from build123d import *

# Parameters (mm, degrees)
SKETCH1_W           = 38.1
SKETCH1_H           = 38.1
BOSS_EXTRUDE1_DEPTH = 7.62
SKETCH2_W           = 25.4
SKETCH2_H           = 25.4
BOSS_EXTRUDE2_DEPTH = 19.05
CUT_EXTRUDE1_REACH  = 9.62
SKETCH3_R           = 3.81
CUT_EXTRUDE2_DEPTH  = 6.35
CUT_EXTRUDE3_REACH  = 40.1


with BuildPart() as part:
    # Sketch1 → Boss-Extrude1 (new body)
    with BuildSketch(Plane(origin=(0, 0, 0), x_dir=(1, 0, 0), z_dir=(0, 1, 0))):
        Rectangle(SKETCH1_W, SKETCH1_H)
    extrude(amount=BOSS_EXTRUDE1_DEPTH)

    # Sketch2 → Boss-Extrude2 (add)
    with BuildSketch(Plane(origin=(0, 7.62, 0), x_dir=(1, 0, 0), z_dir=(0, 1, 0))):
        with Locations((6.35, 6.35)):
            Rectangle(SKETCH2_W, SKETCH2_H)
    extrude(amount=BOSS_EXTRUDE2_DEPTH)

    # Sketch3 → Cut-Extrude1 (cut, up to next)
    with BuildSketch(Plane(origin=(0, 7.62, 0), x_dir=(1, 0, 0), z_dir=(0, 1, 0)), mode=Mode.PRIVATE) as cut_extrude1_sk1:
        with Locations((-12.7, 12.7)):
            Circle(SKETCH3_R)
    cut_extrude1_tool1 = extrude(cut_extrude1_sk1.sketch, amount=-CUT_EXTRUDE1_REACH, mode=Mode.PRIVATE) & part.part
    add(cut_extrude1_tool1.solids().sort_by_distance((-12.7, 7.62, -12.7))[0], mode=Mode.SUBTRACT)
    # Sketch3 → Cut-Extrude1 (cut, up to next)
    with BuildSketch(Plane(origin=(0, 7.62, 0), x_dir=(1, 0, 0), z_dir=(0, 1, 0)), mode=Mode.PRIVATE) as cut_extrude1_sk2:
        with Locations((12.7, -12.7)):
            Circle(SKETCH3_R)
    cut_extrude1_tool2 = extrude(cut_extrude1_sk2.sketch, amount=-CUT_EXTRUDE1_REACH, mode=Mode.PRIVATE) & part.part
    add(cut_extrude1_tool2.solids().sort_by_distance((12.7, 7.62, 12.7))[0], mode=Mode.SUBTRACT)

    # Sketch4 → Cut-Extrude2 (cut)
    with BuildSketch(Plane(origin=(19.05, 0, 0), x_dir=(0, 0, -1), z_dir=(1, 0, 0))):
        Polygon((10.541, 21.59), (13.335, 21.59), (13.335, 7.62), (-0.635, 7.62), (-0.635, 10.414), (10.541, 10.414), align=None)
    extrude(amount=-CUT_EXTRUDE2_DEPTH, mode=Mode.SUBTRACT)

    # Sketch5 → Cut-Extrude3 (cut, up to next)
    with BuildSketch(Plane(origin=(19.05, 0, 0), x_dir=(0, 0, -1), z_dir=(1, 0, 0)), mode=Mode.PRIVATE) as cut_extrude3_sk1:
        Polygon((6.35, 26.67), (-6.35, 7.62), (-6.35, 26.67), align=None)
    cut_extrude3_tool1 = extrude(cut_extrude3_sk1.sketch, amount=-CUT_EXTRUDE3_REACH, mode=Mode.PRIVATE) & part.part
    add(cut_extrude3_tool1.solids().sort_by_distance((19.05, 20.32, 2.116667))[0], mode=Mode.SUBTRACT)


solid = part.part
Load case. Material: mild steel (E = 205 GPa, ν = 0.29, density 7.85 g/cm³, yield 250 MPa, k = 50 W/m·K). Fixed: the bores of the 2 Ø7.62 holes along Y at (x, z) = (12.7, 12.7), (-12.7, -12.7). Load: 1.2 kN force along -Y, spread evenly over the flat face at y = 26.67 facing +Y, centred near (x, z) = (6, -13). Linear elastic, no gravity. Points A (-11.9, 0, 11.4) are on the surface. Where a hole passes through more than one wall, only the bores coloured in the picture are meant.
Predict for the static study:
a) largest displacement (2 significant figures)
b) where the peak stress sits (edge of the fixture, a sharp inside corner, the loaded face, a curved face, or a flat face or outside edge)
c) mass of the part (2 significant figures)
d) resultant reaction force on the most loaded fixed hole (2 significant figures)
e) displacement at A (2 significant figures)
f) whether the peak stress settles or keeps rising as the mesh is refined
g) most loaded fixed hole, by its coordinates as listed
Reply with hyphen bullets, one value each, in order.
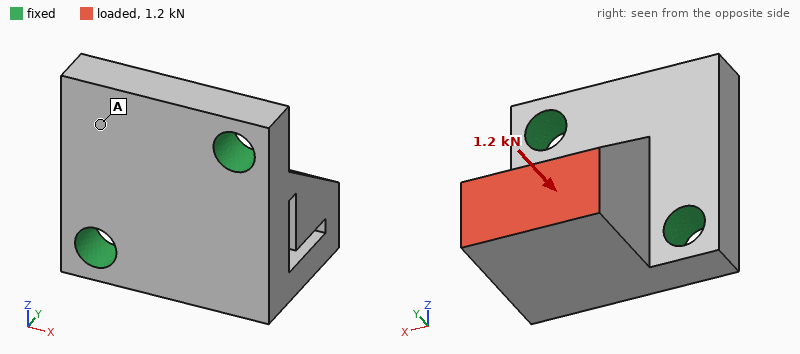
- 9.8 µm
- edge of the fixture
- 150 g
- 810 N
- 2.2 µm
- keeps rising
- (-12.7, -12.7)
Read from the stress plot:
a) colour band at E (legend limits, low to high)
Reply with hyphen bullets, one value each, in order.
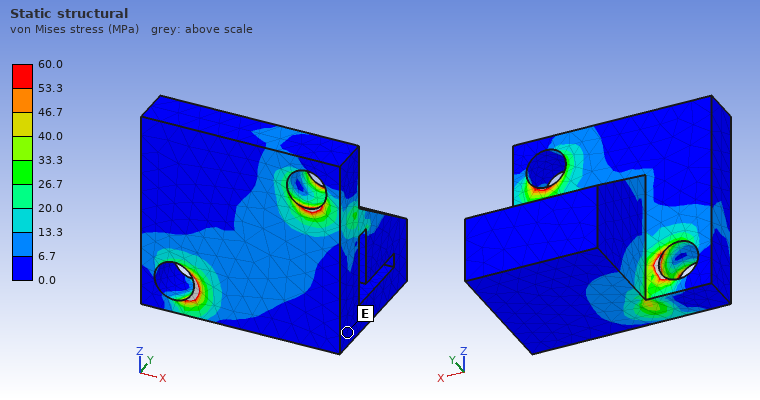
- 0.0 to 6.7 MPa
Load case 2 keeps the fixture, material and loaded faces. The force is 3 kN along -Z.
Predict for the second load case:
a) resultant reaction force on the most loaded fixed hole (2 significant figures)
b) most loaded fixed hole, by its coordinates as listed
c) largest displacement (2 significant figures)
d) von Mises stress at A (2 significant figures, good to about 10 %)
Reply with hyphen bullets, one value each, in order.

- 2.4 kN
- (12.7, 12.7)
- 34 µm
- 26 MPa
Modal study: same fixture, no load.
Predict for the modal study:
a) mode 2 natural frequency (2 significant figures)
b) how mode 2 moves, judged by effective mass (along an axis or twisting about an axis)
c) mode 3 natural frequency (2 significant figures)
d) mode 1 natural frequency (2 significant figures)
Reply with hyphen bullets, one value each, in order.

- 15 kHz
- along Y
- 18 kHz
- 6900 Hz
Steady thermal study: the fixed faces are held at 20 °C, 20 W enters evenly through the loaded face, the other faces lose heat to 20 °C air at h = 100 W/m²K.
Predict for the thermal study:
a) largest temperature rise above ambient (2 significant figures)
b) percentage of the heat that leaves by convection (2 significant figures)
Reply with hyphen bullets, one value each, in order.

- 30 K
- 26 %
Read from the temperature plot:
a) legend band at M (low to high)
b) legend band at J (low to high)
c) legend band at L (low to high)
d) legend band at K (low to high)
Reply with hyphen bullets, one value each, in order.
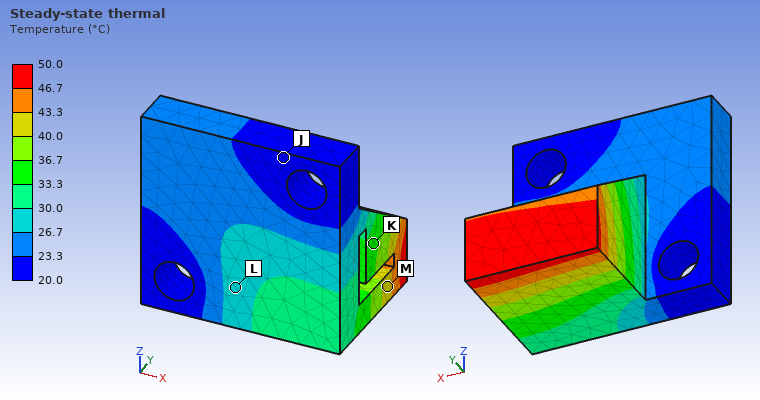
- 40.0 to 43.3 °C
- 20.0 to 23.3 °C
- 26.7 to 30.0 °C
- 33.3 to 36.7 °C
